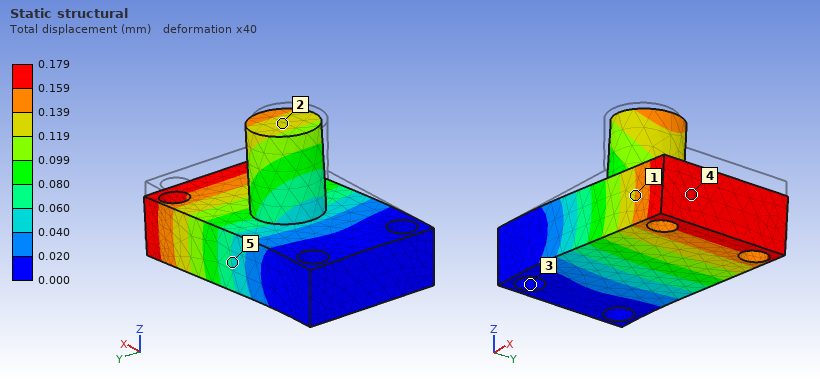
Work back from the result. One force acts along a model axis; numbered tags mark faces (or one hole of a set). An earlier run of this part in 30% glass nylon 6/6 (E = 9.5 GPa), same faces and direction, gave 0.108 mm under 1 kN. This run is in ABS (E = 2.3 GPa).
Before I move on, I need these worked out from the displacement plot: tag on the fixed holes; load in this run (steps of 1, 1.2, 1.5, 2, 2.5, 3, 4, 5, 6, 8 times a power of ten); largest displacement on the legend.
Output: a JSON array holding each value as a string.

["3", "400 N", "0.179 mm"]
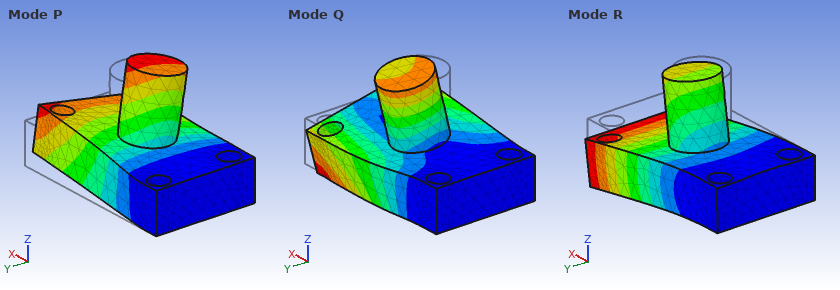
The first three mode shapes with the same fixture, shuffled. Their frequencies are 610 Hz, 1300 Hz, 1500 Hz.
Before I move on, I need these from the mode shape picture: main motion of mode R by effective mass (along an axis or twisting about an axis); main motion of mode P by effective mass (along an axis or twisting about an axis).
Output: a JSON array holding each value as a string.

["along Z", "along Y"]
